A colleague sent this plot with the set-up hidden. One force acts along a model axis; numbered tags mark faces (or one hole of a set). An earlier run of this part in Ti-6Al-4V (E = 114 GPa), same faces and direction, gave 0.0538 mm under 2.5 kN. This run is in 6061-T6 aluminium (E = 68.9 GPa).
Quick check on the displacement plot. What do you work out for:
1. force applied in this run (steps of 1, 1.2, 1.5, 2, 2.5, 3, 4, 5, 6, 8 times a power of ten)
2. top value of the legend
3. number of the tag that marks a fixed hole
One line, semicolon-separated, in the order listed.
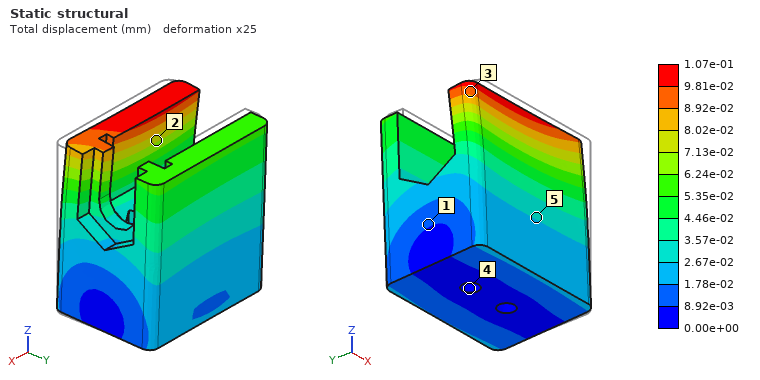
3 kN; 1.07e-01 mm; 4
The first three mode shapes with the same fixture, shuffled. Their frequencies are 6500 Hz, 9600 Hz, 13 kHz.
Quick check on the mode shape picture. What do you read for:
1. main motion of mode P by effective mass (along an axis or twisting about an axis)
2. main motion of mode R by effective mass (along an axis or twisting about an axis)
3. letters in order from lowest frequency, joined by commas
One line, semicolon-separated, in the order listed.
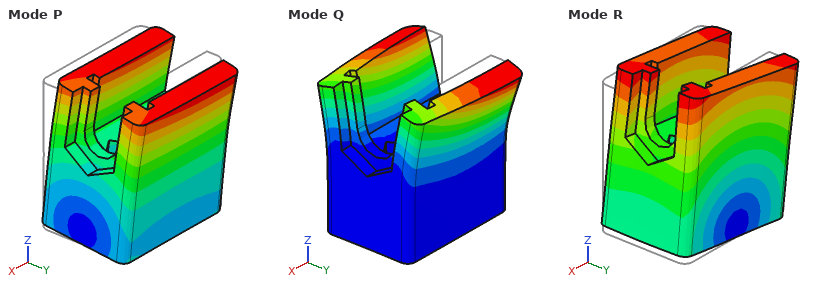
along Y; along X; P, R, Q
